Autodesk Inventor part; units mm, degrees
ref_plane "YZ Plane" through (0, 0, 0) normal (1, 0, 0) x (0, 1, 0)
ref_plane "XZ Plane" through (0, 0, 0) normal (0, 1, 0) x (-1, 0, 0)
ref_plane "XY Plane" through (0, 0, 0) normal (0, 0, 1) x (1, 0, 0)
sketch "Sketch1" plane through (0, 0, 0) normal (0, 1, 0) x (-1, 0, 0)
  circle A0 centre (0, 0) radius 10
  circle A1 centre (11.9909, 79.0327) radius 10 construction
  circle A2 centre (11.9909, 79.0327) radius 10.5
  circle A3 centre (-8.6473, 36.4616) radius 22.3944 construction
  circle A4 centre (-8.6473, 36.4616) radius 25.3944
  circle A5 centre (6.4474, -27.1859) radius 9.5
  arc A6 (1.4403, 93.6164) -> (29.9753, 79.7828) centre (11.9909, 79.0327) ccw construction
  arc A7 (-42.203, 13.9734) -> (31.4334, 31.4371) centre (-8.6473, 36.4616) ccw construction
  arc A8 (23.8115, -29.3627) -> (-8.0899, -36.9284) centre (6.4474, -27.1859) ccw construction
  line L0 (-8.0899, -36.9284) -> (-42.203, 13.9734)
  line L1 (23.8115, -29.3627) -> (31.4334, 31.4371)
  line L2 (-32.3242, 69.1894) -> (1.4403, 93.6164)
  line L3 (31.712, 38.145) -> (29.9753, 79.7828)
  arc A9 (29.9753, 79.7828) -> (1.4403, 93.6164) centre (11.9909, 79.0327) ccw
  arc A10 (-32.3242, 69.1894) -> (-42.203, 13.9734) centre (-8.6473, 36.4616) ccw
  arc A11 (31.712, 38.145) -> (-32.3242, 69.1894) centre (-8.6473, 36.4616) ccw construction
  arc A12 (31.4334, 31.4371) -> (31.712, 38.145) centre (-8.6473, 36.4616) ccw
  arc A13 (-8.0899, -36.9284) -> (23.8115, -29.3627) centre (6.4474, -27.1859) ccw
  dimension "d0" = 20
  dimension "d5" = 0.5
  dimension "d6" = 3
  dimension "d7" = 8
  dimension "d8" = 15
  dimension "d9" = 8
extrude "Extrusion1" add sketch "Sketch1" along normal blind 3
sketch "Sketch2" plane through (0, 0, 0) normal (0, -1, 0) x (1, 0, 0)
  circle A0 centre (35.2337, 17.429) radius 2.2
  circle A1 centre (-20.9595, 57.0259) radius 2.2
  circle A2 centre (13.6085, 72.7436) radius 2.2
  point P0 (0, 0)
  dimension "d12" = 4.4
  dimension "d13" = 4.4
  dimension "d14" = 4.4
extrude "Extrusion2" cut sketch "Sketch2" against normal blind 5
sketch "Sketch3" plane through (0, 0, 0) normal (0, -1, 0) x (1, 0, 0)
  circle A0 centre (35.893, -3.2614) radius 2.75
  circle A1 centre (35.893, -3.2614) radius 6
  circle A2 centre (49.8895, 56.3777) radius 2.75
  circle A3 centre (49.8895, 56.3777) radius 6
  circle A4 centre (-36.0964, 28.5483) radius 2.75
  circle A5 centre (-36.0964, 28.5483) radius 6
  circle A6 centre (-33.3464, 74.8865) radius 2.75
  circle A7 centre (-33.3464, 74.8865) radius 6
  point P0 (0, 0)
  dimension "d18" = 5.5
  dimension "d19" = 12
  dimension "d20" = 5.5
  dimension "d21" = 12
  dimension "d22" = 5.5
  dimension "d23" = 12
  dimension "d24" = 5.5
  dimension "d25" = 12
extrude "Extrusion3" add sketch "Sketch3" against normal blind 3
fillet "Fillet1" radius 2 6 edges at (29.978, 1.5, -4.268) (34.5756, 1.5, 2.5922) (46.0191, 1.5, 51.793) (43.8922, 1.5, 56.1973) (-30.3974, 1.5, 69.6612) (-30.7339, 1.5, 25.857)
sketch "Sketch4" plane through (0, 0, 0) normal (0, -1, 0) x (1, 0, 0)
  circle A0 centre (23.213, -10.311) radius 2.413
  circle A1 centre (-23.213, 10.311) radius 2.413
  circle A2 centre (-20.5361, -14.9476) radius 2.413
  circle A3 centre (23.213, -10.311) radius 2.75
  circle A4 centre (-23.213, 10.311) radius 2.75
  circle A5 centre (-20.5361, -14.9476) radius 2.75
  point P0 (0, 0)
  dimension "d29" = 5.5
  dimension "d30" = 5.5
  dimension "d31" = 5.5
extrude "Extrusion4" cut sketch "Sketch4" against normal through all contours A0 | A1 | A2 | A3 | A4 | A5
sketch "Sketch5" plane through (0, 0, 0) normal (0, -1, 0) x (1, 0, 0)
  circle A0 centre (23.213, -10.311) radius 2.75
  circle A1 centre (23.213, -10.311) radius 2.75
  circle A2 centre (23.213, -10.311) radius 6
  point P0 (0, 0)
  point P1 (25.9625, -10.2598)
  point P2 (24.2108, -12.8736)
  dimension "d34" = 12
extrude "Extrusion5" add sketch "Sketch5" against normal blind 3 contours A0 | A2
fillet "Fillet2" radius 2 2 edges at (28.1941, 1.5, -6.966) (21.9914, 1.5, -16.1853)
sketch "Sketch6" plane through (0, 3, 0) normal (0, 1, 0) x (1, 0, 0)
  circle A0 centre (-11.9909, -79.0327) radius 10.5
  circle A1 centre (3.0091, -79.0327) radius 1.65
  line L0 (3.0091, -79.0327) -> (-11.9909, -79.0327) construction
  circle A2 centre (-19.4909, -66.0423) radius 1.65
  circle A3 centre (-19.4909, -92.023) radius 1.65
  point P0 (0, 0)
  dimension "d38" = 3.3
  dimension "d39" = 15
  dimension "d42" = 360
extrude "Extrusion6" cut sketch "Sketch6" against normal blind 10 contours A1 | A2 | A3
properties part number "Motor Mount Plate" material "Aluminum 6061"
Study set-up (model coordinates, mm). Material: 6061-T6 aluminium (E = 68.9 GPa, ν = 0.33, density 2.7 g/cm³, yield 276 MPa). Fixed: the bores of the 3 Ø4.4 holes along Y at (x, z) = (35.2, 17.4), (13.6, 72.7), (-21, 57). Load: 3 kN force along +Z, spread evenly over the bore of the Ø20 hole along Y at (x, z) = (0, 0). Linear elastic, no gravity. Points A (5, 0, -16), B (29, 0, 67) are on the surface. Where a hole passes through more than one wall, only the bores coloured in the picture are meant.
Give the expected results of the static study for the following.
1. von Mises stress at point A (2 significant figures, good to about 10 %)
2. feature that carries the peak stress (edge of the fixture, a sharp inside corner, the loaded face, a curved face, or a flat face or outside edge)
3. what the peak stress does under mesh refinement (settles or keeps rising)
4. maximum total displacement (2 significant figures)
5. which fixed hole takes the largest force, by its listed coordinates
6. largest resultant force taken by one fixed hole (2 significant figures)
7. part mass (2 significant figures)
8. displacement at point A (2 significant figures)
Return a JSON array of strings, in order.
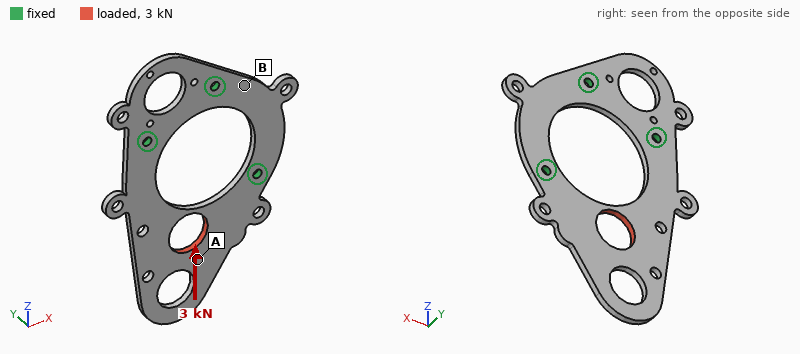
["36 MPa", "edge of the fixture", "keeps rising", "67 µm", "(-21, 57)", "2.0 kN", "44 g", "58 µm"]
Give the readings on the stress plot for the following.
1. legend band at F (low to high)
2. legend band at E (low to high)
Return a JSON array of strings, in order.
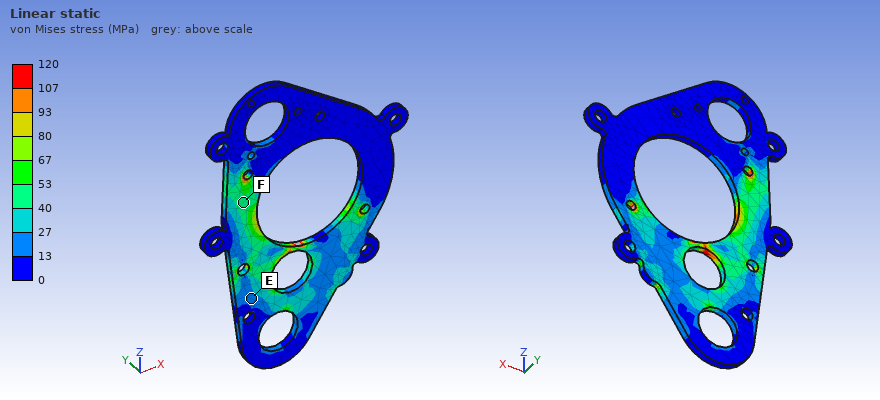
["40 to 53 MPa", "13 to 27 MPa"]
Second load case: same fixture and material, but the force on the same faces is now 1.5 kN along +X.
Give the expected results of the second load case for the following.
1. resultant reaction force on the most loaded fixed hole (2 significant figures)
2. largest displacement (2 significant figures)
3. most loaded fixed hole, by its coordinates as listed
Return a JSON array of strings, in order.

["1.4 kN", "55 µm", "(35.2, 17.4)"]
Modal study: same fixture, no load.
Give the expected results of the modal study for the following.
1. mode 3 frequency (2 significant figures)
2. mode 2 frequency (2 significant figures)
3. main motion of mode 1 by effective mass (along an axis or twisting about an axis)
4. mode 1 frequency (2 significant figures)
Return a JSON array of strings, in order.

["2400 Hz", "1500 Hz", "along Y", "450 Hz"]
